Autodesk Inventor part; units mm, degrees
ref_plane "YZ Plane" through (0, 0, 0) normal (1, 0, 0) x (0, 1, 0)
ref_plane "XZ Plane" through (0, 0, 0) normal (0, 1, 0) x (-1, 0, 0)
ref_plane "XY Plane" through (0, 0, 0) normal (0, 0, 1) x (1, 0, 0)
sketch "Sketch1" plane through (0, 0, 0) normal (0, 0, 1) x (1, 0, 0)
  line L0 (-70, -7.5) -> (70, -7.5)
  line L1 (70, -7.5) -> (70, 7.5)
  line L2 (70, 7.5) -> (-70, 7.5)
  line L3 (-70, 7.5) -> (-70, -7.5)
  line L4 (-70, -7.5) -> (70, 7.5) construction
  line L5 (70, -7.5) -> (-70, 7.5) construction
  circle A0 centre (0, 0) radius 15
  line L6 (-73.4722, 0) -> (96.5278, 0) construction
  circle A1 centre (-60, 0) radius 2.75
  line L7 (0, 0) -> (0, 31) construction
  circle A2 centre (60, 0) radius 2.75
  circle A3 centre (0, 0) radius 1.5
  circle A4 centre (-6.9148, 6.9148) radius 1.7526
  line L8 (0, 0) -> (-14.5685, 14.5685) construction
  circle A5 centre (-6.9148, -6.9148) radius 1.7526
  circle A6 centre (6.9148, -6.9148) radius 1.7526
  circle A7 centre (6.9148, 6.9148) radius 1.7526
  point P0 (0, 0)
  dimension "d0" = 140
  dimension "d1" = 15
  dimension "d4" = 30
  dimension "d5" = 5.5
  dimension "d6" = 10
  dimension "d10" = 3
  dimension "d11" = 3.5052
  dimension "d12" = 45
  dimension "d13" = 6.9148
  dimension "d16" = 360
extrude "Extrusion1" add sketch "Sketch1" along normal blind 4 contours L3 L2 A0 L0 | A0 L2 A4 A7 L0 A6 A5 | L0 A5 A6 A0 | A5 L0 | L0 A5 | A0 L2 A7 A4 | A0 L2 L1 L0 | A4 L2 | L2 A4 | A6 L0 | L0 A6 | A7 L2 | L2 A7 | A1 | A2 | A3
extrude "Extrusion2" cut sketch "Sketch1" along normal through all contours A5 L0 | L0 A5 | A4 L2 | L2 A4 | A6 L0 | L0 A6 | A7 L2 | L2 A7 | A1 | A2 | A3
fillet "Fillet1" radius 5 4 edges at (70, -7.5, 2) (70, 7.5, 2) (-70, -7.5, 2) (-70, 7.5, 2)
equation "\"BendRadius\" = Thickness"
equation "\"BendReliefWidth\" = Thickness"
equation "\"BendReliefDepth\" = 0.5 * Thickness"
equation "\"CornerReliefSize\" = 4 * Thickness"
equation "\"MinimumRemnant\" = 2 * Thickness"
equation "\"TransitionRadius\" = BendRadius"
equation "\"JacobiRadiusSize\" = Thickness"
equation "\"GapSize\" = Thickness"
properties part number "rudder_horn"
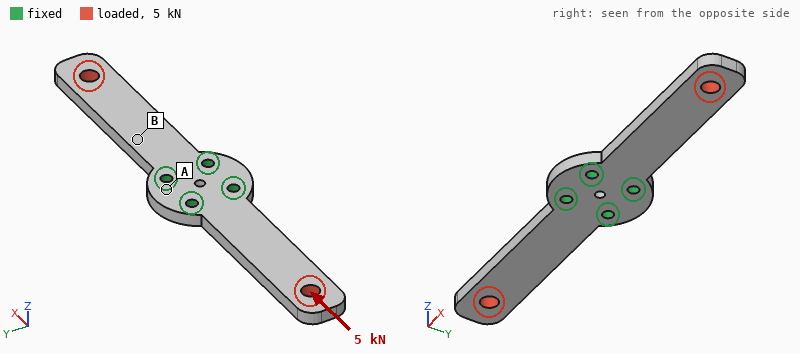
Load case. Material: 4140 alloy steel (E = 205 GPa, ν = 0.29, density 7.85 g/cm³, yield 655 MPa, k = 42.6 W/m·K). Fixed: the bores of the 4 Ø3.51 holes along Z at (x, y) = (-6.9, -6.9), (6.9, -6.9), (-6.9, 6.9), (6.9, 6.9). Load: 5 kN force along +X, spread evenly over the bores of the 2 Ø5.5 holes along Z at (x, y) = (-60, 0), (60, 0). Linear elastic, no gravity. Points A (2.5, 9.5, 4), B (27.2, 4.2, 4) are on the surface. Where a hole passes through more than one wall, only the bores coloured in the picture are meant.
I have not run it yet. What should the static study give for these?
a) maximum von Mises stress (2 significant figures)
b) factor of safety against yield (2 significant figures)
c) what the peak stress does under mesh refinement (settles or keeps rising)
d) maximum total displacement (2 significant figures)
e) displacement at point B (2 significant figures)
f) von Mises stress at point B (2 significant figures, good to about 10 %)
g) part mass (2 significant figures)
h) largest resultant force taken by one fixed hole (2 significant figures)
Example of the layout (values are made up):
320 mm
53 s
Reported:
100 MPa
6.5
settles
12 µm
4.1 µm
42 MPa
71 g
1.3 kN
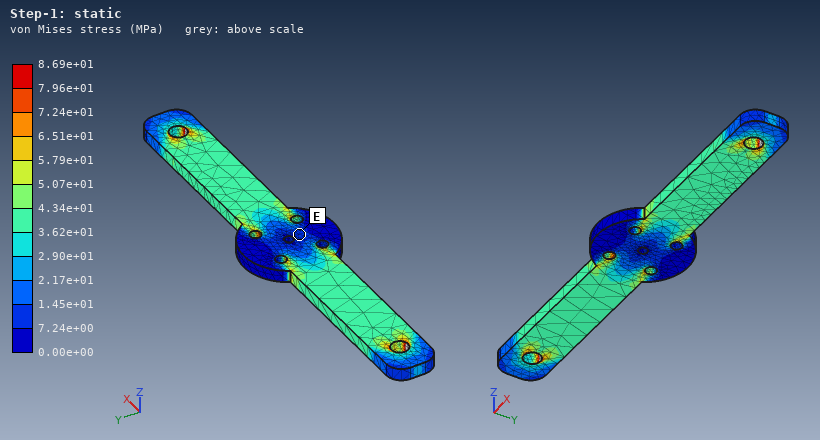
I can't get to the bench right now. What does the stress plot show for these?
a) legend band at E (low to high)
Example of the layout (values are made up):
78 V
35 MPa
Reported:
7.24e+00 to 1.45e+01 MPa
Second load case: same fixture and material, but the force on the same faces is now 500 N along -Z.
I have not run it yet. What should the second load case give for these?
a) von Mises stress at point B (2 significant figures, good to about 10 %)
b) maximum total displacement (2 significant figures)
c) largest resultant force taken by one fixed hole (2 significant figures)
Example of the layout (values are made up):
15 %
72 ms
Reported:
200 MPa
0.91 mm
130 N
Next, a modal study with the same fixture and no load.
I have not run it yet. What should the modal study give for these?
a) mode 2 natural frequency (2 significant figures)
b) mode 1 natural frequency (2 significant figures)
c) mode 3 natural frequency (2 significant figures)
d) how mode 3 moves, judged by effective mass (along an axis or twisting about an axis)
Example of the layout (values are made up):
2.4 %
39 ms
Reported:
910 Hz
910 Hz
3400 Hz
twisting about Z
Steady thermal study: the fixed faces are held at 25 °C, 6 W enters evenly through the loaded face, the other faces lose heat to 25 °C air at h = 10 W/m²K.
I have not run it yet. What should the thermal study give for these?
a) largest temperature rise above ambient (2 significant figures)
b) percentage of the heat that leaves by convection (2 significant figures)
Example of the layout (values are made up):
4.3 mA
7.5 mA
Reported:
54 K
22 %
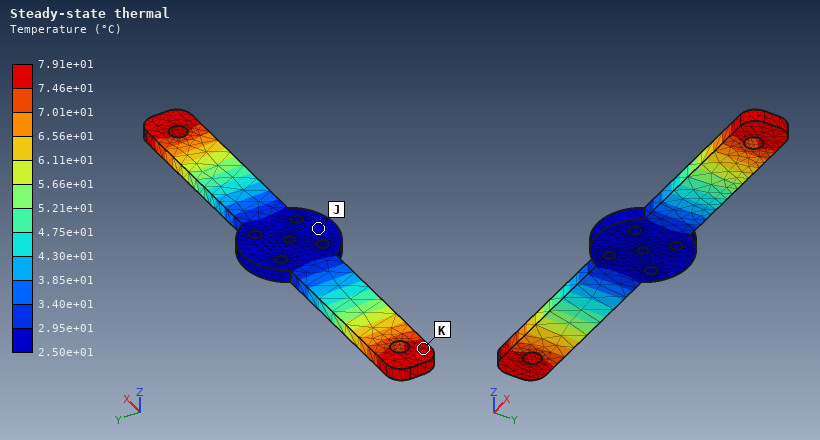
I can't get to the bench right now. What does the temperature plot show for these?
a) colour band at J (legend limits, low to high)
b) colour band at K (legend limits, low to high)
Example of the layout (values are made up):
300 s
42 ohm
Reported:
2.50e+01 to 2.95e+01 °C
7.46e+01 to 7.91e+01 °C
